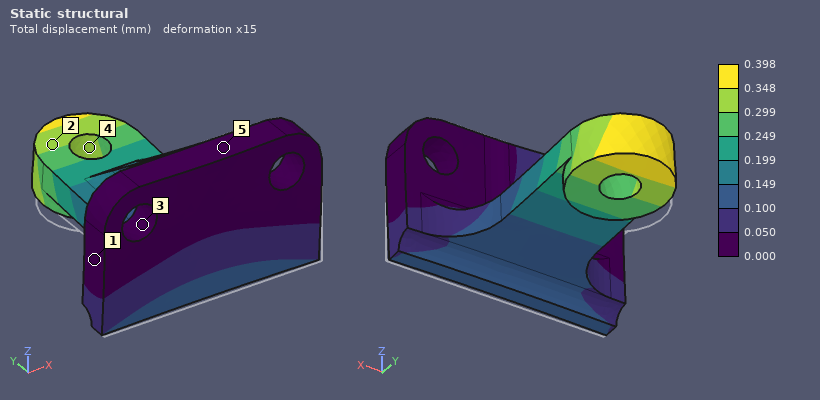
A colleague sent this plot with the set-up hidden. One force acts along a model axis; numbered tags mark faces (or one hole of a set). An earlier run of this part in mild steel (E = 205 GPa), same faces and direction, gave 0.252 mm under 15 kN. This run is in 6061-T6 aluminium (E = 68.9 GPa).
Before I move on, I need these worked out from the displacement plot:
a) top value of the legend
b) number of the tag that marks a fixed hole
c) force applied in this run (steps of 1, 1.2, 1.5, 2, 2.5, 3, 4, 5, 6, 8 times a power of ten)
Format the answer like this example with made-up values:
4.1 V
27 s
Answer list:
0.398 mm
3
8 kN
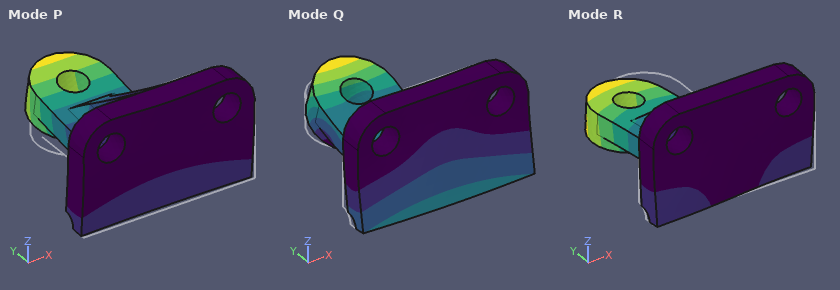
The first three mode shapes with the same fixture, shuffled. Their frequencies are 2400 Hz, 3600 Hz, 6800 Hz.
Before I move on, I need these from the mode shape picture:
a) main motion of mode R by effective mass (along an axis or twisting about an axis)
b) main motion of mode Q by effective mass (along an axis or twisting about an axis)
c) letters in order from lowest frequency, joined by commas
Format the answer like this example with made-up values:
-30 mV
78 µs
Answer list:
along X
along Y
P, R, Q
